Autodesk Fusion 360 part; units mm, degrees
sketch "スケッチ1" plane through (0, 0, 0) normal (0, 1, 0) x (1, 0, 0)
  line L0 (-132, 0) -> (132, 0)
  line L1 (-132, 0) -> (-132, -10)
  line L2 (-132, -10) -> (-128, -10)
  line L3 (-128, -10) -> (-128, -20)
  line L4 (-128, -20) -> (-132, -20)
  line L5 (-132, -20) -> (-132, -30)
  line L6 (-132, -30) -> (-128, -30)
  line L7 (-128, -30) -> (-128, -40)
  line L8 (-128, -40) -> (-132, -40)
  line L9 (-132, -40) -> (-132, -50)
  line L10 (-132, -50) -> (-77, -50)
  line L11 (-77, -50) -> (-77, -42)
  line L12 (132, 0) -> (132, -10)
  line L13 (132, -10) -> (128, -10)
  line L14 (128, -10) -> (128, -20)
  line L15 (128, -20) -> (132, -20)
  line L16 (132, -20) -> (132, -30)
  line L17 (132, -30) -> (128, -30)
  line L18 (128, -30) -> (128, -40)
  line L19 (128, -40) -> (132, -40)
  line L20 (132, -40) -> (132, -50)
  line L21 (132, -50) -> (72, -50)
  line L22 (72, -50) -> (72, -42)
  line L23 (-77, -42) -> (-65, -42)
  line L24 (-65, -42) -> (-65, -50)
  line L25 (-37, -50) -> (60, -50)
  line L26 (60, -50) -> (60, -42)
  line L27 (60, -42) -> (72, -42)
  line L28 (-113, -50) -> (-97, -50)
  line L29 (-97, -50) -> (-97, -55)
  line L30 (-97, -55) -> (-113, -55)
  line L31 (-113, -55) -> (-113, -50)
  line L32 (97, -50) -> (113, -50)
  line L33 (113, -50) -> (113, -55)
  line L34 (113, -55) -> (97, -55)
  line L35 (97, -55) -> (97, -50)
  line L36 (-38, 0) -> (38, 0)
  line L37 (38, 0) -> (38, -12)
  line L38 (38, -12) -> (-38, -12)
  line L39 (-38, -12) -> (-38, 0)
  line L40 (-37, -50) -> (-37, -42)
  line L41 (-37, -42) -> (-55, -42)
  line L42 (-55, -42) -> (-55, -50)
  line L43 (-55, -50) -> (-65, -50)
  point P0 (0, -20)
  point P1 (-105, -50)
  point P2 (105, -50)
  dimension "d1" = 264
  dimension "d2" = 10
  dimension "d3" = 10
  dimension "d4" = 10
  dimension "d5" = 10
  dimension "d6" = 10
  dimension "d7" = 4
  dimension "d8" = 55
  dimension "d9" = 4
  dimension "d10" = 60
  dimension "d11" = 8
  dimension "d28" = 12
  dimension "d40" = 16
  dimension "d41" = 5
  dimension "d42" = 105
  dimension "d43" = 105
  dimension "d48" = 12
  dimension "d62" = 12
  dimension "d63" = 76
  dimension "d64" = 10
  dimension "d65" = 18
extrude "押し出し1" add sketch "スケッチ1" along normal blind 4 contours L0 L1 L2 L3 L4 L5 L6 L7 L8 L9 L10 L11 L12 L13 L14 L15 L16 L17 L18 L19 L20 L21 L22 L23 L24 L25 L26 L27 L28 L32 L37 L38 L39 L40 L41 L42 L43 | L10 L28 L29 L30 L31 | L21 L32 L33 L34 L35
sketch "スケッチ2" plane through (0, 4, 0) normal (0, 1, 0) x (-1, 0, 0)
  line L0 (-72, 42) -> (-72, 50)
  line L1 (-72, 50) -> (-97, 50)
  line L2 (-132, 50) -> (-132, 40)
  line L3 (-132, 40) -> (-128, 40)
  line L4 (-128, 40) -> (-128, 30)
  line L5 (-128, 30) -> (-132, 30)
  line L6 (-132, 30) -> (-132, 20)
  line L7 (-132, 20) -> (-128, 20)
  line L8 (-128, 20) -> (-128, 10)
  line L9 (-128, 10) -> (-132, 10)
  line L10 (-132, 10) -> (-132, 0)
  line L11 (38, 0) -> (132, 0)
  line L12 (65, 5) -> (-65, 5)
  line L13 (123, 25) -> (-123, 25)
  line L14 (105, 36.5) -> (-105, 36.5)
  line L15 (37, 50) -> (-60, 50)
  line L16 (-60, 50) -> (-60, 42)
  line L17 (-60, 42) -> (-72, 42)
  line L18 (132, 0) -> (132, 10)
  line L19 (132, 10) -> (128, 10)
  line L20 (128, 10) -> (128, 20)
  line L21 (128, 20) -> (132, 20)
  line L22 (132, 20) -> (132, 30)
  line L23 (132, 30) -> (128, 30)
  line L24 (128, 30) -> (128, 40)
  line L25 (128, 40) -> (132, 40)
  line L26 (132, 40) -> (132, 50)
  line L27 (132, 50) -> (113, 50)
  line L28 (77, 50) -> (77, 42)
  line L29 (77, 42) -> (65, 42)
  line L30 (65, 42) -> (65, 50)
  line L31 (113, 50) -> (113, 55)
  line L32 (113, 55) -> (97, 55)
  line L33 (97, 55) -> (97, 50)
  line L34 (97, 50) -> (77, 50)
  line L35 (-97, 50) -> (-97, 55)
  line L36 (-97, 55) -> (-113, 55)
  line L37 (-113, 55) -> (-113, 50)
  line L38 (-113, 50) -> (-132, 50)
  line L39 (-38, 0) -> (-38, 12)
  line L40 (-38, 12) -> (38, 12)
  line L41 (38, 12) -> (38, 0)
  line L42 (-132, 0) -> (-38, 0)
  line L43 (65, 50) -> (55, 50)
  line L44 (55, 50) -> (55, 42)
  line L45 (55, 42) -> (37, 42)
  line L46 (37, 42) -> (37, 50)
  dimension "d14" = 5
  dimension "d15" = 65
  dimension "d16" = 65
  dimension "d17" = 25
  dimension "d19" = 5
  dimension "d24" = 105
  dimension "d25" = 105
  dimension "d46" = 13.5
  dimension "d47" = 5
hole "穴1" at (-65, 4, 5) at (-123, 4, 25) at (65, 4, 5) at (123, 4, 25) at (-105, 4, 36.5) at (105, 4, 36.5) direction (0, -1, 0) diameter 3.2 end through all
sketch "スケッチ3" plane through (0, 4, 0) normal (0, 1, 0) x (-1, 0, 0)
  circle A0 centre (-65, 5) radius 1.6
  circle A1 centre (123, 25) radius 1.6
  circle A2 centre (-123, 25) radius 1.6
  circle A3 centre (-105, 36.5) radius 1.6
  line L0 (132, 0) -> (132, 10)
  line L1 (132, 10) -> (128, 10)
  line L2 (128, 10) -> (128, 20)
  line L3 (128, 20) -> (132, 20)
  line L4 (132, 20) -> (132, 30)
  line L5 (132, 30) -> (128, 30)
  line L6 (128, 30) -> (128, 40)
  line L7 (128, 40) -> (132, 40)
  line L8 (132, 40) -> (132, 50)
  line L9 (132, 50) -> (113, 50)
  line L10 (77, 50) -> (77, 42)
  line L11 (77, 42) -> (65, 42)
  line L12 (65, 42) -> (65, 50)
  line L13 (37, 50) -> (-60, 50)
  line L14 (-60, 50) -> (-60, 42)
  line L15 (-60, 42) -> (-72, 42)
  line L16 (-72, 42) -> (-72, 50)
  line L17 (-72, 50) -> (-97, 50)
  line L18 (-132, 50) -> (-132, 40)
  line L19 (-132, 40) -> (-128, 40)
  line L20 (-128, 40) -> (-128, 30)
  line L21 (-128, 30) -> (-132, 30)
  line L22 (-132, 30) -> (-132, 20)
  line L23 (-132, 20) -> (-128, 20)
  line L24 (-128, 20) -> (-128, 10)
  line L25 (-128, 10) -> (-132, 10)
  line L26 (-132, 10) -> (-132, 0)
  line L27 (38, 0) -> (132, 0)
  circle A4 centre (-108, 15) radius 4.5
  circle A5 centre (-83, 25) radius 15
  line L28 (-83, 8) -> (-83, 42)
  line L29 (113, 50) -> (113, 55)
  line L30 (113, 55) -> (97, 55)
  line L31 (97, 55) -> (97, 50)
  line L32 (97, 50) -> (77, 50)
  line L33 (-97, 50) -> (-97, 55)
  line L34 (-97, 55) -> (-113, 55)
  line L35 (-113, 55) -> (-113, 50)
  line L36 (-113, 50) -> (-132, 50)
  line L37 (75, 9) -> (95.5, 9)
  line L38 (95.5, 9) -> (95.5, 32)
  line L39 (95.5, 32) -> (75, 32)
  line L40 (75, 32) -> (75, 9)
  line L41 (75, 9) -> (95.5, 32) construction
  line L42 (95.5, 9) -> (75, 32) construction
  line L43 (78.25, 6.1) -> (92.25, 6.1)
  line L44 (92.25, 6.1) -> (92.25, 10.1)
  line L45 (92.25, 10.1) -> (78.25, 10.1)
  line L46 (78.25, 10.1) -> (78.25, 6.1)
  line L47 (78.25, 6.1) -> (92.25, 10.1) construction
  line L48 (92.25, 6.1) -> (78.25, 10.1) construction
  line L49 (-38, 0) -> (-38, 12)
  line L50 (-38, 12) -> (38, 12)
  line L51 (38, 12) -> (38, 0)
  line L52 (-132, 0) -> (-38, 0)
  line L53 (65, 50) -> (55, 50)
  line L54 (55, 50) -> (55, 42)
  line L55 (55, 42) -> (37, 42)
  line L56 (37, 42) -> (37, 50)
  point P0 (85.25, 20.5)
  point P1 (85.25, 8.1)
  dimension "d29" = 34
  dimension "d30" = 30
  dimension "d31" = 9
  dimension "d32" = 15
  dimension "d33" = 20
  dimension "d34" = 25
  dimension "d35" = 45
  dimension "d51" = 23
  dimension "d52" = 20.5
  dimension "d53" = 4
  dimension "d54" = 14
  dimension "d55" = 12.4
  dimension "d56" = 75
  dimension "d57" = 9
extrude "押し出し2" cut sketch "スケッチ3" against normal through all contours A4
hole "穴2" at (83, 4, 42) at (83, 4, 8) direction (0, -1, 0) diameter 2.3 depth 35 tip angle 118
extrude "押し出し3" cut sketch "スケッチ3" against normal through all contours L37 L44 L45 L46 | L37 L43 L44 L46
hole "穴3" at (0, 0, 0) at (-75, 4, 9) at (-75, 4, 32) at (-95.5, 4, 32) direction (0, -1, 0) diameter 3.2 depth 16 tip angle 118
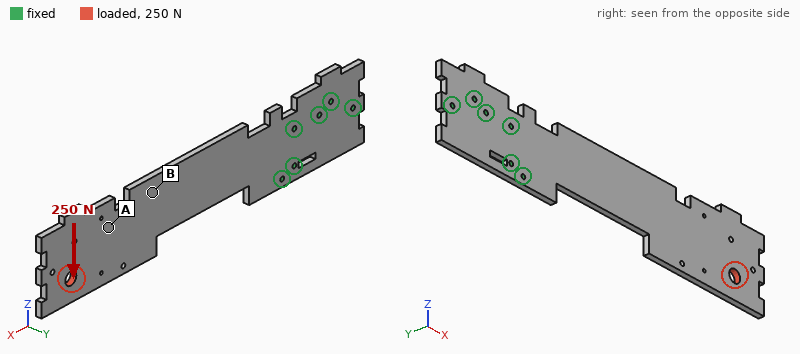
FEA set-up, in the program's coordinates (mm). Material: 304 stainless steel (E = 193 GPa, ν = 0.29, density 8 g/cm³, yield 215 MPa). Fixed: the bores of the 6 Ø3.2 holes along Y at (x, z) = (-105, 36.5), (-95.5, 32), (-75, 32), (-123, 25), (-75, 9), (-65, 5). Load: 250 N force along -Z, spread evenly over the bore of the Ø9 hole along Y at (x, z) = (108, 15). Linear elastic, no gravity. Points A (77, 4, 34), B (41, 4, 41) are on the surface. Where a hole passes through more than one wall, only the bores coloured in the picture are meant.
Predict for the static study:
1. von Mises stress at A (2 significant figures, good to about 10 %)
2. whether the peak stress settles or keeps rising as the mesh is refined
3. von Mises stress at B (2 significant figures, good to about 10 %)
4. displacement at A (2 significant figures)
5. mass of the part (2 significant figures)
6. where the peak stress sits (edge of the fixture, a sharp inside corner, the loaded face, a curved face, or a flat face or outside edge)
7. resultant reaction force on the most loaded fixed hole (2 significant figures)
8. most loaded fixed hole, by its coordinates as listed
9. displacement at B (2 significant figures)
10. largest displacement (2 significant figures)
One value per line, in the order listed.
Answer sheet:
5.2 MPa
keeps rising
11 MPa
0.12 mm
380 g
edge of the fixture
1.3 kN
(-65, 5)
0.076 mm
0.19 mm
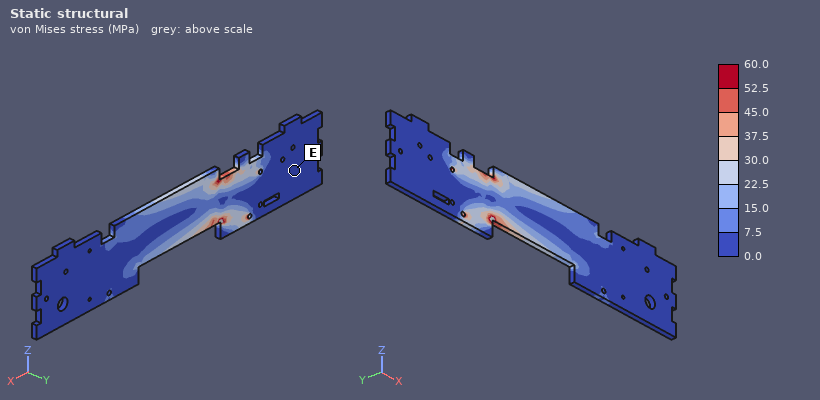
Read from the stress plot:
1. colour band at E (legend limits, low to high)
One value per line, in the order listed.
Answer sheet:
0.0 to 7.5 MPa
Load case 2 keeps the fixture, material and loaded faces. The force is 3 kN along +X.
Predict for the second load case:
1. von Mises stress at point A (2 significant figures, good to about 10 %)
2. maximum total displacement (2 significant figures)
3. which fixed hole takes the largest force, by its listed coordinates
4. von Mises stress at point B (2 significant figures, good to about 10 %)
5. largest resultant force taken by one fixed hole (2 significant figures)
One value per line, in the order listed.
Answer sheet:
8.8 MPa
0.23 mm
(-65, 5)
9.5 MPa
1.4 kN
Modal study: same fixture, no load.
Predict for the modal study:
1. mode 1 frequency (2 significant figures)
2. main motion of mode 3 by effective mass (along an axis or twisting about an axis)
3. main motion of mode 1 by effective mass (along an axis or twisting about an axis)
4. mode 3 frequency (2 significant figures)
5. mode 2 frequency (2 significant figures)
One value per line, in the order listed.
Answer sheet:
70 Hz
twisting about X
along Y
560 Hz
470 Hz
